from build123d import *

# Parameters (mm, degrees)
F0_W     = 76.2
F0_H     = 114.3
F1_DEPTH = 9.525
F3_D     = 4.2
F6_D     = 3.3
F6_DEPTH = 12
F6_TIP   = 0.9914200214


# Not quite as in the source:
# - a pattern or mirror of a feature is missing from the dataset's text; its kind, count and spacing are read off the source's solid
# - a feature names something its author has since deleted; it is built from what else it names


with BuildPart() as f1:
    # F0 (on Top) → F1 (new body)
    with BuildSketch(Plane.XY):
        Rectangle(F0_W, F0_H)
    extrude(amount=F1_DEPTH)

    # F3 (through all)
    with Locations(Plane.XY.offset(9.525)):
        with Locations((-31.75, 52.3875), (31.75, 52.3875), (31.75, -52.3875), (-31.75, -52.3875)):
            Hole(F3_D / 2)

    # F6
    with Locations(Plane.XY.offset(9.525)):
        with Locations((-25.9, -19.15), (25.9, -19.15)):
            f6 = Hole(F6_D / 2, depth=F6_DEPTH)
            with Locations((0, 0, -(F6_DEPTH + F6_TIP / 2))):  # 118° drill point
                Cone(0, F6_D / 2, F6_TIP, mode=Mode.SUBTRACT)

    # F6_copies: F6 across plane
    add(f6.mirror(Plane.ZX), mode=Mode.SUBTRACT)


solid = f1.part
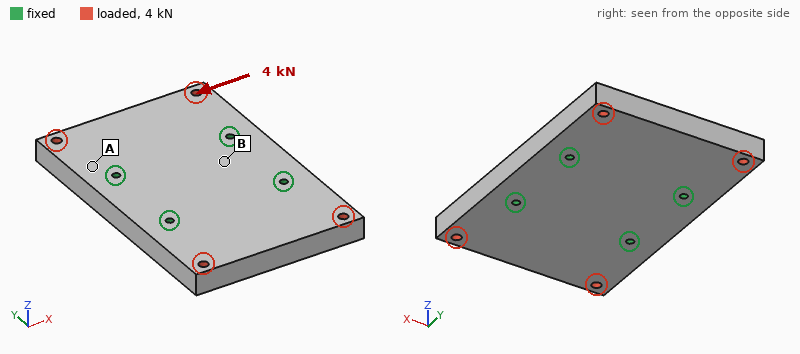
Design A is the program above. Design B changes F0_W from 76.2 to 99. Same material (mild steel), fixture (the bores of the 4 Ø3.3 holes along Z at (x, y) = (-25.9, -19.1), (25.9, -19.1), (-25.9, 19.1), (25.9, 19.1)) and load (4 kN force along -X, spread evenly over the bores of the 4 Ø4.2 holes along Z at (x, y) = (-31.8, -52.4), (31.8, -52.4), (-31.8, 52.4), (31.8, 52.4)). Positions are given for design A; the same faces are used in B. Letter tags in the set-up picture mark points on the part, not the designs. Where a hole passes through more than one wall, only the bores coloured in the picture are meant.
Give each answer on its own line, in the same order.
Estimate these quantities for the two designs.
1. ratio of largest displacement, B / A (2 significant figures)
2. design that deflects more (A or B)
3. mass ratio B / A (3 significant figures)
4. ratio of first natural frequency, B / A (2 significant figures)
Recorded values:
0.73
A
1.30
0.97
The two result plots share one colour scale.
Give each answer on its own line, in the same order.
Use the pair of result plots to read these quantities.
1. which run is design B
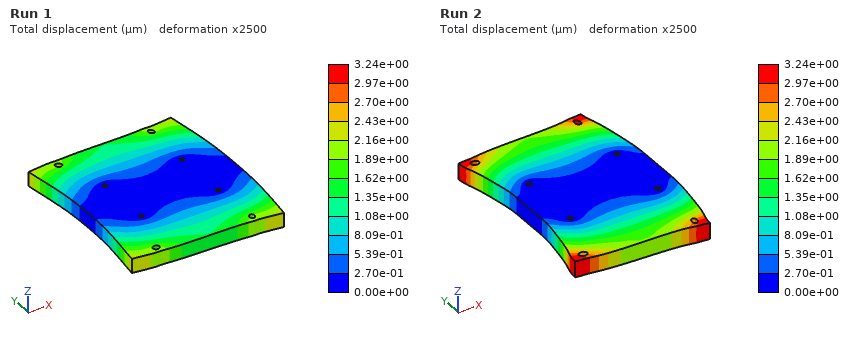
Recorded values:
Run 1
